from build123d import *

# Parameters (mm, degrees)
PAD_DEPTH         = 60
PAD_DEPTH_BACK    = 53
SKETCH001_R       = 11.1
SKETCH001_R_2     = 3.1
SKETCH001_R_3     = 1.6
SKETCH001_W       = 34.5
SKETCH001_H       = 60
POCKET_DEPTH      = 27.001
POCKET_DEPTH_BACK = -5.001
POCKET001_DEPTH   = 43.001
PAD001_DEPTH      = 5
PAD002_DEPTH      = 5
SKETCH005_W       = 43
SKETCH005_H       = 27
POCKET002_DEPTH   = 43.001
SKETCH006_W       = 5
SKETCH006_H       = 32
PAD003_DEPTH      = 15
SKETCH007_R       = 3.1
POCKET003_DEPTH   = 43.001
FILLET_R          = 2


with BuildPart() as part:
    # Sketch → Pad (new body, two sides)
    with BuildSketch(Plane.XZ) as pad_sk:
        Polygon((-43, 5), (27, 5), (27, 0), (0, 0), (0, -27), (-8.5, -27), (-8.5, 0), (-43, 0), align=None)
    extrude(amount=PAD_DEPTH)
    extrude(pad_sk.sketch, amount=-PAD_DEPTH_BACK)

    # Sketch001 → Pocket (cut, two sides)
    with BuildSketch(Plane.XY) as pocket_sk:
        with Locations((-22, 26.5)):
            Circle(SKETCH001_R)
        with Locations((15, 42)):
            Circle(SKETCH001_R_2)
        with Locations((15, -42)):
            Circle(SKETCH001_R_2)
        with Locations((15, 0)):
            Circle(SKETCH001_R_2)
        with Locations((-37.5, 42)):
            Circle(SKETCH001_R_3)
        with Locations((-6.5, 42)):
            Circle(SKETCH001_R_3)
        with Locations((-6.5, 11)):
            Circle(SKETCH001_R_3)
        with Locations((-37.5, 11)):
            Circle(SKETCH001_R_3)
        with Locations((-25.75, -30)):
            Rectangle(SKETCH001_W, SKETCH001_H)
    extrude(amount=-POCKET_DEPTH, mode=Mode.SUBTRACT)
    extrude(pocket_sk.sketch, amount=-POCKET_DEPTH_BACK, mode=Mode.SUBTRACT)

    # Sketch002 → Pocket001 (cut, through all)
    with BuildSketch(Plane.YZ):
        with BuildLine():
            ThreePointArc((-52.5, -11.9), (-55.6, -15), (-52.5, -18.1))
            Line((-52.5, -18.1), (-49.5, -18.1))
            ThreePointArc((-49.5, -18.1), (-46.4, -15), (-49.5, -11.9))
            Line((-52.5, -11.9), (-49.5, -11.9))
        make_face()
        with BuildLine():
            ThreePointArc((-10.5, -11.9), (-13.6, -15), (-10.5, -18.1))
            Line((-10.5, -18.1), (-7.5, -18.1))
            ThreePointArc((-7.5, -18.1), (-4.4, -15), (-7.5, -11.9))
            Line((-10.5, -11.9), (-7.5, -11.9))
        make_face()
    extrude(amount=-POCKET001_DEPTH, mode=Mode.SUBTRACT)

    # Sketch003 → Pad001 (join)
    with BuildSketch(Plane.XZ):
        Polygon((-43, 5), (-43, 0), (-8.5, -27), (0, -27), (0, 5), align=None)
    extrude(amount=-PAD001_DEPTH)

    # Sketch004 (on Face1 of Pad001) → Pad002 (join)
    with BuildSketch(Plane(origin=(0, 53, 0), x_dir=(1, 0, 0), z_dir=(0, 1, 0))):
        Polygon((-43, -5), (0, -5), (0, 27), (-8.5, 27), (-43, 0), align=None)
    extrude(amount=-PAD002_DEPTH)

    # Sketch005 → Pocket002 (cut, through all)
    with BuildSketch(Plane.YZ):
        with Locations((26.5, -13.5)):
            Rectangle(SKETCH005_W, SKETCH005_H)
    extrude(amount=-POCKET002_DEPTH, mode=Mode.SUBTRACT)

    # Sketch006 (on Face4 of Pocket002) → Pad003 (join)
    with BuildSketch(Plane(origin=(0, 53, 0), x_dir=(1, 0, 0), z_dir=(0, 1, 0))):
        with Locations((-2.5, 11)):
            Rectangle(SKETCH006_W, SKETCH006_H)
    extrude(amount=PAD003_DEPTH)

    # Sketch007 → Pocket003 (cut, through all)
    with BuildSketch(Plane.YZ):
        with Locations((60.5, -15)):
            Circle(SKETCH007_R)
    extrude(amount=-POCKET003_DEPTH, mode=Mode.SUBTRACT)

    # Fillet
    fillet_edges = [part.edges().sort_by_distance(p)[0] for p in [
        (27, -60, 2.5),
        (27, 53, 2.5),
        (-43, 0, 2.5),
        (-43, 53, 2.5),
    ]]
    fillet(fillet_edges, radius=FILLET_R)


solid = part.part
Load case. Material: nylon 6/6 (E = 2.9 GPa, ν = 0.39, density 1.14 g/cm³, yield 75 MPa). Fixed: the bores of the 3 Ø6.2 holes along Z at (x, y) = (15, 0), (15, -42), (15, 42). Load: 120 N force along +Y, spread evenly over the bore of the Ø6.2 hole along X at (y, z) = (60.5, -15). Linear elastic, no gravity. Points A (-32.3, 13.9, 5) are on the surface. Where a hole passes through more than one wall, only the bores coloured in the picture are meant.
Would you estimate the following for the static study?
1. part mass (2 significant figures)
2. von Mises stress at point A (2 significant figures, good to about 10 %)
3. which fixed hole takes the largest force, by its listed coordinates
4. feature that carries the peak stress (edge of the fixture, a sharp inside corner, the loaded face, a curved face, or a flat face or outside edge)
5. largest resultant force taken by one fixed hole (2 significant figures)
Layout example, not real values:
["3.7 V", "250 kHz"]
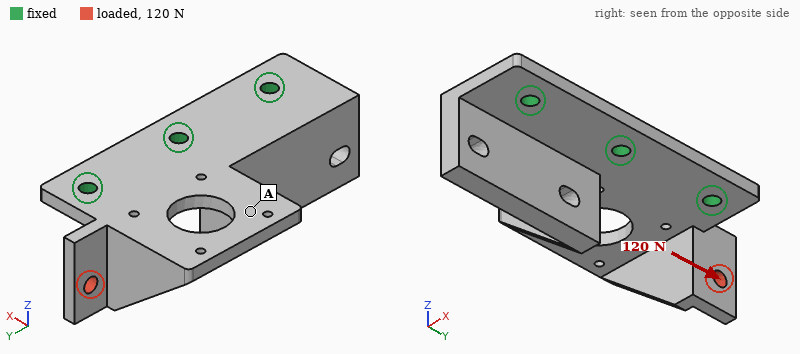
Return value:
["56 g", "3.2 MPa", "(15, 42)", "a curved face", "79 N"]
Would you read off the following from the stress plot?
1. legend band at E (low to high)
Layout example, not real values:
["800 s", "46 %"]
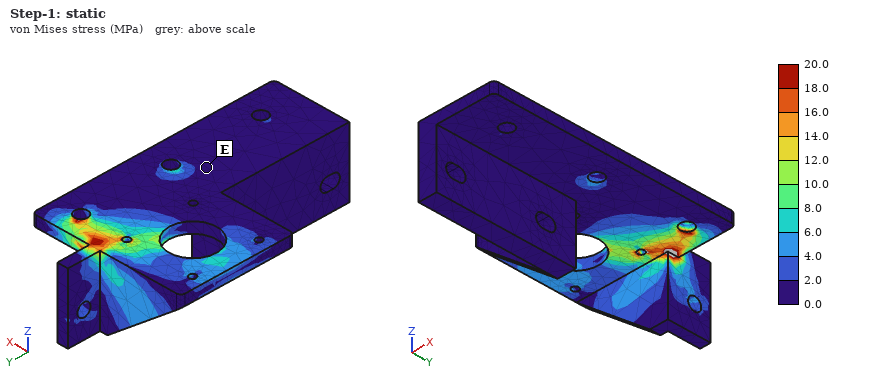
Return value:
["0.0 to 2.0 MPa"]
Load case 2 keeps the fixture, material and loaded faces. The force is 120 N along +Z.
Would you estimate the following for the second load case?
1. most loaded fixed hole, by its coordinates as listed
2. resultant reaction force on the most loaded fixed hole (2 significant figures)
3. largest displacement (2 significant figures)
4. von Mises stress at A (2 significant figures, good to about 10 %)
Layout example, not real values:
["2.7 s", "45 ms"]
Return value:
["(15, 42)", "140 N", "1.6 mm", "4.9 MPa"]
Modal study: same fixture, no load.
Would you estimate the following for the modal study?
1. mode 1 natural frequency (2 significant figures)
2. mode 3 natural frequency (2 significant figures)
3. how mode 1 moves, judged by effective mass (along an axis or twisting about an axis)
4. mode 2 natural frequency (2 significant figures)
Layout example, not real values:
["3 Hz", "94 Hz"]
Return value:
["410 Hz", "920 Hz", "along Z", "600 Hz"]
